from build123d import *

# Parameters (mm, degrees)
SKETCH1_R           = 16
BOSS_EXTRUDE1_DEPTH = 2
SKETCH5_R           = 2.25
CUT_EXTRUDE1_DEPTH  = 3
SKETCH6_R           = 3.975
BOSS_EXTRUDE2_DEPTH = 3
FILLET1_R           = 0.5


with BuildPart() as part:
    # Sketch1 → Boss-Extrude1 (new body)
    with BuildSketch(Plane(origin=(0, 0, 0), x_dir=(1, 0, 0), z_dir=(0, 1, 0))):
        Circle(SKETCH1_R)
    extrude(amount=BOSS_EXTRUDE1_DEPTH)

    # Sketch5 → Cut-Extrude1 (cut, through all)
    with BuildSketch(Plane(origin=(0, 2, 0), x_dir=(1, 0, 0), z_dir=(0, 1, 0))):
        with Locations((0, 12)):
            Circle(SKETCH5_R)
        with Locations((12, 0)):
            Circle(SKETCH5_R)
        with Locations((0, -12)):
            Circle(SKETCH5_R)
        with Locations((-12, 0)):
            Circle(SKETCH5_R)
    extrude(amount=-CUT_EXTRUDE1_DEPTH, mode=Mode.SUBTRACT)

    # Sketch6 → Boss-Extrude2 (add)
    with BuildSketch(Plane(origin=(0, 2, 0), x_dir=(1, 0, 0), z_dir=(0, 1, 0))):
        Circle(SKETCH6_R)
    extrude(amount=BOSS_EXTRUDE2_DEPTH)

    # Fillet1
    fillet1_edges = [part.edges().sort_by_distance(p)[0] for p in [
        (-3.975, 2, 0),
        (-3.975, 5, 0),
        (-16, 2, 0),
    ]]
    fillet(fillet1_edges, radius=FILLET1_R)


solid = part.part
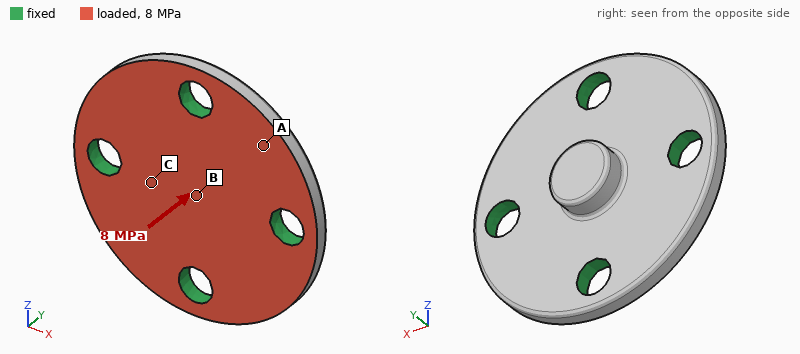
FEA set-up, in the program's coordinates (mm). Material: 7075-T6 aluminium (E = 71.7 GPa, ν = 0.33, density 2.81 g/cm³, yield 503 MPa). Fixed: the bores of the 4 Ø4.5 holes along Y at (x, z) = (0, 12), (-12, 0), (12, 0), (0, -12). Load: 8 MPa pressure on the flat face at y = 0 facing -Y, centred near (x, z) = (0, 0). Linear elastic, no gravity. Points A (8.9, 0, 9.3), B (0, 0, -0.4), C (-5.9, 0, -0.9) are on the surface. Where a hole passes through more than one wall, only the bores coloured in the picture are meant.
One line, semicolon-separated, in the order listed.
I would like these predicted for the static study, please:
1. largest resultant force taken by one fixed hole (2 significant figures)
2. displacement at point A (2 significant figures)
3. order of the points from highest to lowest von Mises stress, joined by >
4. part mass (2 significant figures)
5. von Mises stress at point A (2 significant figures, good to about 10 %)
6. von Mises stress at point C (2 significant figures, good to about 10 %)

1.5 kN; 37 µm; A > C > B; 4.6 g; 110 MPa; 57 MPa
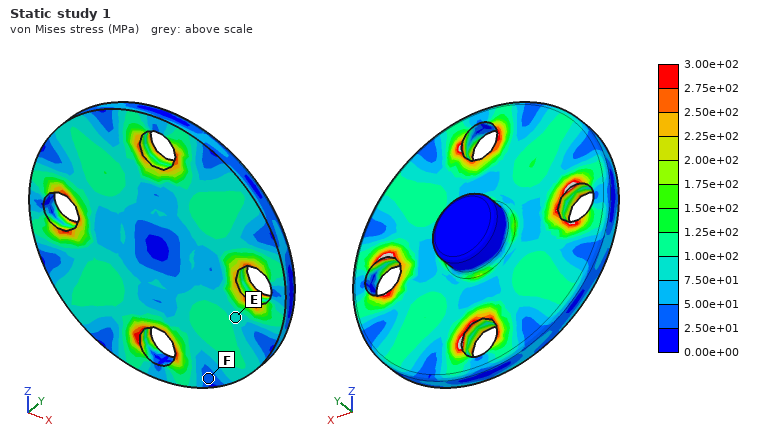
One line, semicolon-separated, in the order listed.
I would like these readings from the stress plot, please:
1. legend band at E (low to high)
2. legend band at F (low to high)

7.50e+01 to 1.00e+02 MPa; 2.50e+01 to 5.00e+01 MPa
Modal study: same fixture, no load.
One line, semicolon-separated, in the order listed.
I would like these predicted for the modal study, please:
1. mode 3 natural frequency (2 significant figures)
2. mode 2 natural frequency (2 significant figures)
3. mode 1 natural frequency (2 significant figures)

33 kHz; 33 kHz; 32 kHz
